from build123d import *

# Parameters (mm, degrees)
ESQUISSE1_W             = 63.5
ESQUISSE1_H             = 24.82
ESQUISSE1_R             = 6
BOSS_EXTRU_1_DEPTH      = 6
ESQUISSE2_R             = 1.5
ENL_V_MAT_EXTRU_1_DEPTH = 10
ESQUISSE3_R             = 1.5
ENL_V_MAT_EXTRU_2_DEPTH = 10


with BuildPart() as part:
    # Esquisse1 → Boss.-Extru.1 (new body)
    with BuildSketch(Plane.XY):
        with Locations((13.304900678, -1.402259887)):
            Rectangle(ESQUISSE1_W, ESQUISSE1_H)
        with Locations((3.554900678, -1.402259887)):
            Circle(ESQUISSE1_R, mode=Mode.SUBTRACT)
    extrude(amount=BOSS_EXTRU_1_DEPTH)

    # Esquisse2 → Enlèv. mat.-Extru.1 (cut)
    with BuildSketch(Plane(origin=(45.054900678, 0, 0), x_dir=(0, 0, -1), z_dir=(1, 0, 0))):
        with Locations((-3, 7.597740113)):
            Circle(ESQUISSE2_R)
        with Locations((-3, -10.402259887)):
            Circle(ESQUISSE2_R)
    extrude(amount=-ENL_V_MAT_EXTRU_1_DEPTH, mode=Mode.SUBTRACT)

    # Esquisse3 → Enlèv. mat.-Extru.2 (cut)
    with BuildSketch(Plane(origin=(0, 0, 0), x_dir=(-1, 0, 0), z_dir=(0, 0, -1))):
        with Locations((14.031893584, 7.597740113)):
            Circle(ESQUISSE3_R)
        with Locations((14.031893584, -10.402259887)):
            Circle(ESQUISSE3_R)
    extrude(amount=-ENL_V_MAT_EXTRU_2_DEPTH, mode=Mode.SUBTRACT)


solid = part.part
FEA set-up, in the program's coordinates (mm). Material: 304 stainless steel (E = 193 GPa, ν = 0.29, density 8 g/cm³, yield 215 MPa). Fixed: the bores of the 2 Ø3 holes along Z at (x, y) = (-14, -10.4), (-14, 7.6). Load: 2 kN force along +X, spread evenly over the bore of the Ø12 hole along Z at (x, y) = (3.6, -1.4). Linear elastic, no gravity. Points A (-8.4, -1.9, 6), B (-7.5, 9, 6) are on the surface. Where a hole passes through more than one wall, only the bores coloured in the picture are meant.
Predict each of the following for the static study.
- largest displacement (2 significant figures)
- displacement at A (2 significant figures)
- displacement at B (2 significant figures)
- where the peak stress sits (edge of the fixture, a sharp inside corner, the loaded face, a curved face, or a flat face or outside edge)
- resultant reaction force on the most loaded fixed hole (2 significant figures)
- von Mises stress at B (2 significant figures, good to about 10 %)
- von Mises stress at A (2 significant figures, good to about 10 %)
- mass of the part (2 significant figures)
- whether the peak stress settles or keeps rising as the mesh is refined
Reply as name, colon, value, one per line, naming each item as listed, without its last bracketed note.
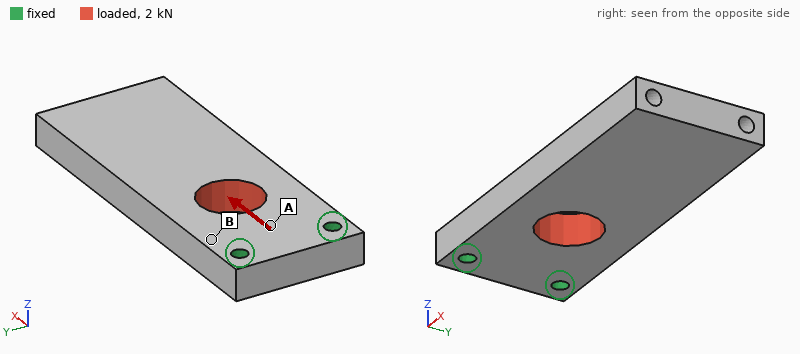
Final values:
largest displacement: 2.4 µm
displacement at A: 0.69 µm
displacement at B: 0.63 µm
where the peak stress sits: edge of the fixture
resultant reaction force on the most loaded fixed hole: 1.0 kN
von Mises stress at B: 18 MPa
von Mises stress at A: 5.6 MPa
mass of the part: 68 g
whether the peak stress settles or keeps rising as the mesh is refined: keeps rising
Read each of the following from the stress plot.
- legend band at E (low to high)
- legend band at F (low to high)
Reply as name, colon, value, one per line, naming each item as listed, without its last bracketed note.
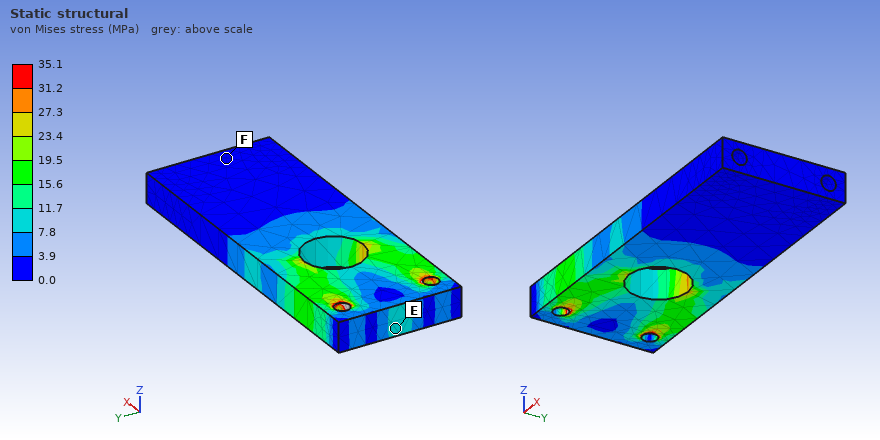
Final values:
legend band at E: 7.8 to 11.7 MPa
legend band at F: 0.0 to 3.9 MPa
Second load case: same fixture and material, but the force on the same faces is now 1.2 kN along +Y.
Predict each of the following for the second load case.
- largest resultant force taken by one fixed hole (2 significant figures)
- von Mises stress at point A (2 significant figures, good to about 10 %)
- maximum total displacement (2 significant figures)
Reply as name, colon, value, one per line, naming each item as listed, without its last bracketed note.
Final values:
largest resultant force taken by one fixed hole: 1.2 kN
von Mises stress at point A: 26 MPa
maximum total displacement: 12 µm
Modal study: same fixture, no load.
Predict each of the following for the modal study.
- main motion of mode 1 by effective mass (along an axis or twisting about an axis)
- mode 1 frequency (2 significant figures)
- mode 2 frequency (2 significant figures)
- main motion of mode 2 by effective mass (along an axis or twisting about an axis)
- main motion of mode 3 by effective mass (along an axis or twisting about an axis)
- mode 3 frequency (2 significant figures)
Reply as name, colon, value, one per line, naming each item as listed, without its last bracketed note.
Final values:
main motion of mode 1 by effective mass: along Z
mode 1 frequency: 1200 Hz
mode 2 frequency: 4700 Hz
main motion of mode 2 by effective mass: along Y
main motion of mode 3 by effective mass: twisting about X
mode 3 frequency: 5600 Hz
